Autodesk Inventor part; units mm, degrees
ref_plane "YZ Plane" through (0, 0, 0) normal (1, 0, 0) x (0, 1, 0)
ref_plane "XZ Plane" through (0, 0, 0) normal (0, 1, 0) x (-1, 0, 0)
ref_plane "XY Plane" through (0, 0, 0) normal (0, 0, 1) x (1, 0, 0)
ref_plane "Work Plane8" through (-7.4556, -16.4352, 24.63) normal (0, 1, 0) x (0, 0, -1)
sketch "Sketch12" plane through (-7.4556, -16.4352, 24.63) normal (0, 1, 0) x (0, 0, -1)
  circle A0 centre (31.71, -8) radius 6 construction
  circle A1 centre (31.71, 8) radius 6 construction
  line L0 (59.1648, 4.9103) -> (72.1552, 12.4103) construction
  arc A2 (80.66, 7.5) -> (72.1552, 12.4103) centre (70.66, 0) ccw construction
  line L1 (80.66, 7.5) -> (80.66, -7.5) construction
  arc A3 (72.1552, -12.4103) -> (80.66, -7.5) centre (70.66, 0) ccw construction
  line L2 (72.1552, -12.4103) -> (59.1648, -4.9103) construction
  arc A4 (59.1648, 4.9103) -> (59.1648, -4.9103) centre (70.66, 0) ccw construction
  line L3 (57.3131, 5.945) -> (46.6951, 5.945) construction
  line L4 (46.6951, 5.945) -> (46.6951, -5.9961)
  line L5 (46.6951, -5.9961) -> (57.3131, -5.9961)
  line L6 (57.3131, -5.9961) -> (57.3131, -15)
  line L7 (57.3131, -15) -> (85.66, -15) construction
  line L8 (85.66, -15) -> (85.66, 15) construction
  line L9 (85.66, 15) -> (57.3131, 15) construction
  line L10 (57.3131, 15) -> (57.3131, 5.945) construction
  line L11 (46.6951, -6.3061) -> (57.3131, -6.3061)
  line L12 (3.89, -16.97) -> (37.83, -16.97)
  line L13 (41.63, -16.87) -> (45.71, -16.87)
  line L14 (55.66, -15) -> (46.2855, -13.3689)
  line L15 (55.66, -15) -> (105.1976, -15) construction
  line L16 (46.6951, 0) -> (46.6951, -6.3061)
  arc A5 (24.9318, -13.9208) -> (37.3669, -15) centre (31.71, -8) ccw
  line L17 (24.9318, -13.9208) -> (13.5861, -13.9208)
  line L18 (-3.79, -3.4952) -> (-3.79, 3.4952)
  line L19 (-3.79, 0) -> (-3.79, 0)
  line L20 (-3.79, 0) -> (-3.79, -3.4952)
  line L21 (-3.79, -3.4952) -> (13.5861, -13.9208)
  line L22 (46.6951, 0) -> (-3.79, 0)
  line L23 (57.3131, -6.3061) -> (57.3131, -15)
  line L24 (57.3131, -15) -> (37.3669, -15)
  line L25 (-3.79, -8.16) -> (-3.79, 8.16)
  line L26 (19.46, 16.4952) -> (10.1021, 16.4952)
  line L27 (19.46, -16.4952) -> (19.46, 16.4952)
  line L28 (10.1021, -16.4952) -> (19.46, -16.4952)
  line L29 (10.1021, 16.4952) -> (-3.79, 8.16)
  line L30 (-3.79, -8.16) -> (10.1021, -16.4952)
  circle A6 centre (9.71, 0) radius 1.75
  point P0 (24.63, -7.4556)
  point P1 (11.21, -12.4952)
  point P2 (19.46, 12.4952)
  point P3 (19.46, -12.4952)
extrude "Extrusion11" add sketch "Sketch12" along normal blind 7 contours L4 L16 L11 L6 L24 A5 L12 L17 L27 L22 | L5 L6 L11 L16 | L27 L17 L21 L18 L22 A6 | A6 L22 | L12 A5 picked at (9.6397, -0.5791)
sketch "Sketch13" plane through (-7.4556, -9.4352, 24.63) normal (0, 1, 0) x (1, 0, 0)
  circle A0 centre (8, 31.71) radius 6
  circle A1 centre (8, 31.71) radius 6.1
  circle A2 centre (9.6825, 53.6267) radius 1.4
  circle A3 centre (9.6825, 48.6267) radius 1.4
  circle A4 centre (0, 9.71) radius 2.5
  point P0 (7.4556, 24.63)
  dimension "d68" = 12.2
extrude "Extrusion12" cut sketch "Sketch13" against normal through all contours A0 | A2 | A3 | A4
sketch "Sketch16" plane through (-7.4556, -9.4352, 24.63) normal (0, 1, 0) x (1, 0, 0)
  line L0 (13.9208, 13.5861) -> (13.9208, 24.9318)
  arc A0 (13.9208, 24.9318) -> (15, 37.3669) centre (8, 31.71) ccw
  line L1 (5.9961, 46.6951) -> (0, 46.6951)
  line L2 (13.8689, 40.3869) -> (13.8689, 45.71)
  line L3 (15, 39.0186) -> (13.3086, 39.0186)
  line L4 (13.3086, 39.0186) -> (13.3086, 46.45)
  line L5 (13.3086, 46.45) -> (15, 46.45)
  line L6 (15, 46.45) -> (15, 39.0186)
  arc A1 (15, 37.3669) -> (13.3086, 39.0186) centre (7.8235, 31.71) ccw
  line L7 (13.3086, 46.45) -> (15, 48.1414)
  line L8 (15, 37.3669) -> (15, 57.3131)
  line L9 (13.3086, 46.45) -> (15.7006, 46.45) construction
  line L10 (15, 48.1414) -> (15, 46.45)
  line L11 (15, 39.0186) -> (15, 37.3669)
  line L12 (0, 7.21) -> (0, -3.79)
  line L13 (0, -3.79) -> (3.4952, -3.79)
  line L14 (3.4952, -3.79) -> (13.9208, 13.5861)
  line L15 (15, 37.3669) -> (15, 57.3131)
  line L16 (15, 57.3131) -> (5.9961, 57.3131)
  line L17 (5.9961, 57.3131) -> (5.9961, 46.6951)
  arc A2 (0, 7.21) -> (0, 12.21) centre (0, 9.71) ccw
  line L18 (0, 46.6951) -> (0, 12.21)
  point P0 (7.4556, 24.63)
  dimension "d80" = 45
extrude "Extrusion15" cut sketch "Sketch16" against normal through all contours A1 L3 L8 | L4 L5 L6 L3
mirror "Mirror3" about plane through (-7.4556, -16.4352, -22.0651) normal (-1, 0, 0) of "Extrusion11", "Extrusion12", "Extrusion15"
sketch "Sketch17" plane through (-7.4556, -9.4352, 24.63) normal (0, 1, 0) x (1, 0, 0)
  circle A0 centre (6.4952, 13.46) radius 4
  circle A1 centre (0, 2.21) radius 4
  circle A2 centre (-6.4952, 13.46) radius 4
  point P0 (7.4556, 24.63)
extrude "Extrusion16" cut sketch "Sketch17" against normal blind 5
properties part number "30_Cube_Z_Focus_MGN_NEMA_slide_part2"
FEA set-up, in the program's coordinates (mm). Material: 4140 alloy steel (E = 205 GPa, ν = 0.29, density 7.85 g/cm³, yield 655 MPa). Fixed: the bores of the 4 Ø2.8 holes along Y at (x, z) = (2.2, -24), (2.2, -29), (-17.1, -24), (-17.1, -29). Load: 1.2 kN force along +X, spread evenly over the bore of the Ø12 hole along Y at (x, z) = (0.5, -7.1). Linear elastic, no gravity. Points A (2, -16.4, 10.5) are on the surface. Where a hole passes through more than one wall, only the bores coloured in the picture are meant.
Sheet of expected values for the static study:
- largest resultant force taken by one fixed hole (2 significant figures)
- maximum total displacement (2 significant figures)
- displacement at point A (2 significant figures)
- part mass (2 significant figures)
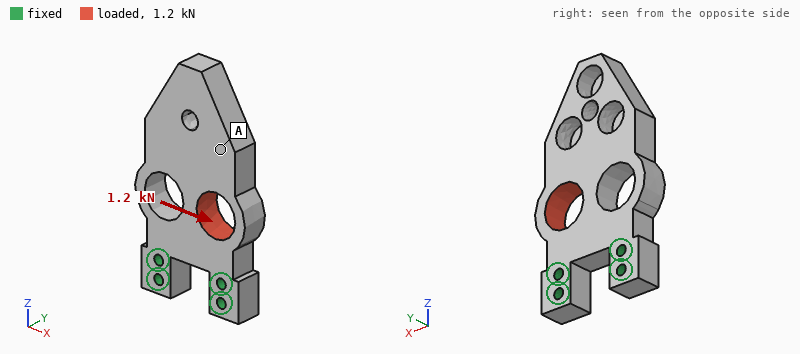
1.0 kN
15 µm
11 µm
60 g
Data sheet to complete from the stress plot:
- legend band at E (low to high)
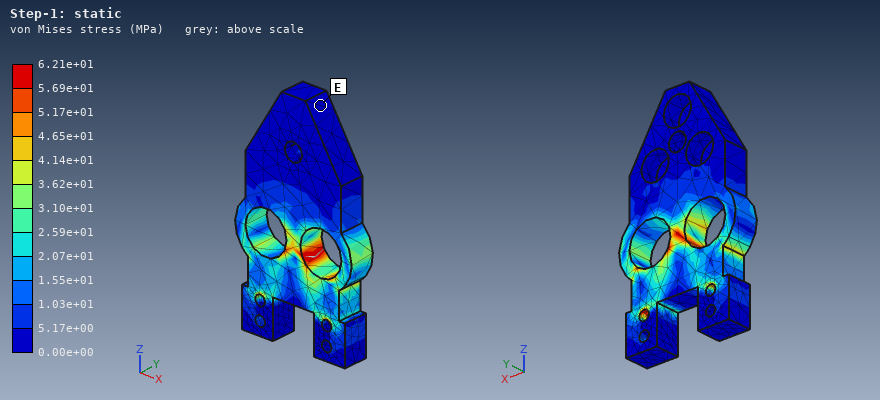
0.00e+00 to 5.17e+00 MPa
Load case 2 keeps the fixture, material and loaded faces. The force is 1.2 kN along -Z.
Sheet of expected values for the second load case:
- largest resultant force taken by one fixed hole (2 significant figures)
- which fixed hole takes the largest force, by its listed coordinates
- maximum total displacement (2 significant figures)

950 N
(2.2, -24)
8.1 µm
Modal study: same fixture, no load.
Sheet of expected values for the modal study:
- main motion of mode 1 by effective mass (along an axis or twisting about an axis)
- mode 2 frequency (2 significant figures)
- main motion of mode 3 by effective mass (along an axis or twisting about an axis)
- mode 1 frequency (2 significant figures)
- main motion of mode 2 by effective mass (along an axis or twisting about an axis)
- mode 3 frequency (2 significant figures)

along Y
5700 Hz
twisting about Z
2100 Hz
along X
8200 Hz
